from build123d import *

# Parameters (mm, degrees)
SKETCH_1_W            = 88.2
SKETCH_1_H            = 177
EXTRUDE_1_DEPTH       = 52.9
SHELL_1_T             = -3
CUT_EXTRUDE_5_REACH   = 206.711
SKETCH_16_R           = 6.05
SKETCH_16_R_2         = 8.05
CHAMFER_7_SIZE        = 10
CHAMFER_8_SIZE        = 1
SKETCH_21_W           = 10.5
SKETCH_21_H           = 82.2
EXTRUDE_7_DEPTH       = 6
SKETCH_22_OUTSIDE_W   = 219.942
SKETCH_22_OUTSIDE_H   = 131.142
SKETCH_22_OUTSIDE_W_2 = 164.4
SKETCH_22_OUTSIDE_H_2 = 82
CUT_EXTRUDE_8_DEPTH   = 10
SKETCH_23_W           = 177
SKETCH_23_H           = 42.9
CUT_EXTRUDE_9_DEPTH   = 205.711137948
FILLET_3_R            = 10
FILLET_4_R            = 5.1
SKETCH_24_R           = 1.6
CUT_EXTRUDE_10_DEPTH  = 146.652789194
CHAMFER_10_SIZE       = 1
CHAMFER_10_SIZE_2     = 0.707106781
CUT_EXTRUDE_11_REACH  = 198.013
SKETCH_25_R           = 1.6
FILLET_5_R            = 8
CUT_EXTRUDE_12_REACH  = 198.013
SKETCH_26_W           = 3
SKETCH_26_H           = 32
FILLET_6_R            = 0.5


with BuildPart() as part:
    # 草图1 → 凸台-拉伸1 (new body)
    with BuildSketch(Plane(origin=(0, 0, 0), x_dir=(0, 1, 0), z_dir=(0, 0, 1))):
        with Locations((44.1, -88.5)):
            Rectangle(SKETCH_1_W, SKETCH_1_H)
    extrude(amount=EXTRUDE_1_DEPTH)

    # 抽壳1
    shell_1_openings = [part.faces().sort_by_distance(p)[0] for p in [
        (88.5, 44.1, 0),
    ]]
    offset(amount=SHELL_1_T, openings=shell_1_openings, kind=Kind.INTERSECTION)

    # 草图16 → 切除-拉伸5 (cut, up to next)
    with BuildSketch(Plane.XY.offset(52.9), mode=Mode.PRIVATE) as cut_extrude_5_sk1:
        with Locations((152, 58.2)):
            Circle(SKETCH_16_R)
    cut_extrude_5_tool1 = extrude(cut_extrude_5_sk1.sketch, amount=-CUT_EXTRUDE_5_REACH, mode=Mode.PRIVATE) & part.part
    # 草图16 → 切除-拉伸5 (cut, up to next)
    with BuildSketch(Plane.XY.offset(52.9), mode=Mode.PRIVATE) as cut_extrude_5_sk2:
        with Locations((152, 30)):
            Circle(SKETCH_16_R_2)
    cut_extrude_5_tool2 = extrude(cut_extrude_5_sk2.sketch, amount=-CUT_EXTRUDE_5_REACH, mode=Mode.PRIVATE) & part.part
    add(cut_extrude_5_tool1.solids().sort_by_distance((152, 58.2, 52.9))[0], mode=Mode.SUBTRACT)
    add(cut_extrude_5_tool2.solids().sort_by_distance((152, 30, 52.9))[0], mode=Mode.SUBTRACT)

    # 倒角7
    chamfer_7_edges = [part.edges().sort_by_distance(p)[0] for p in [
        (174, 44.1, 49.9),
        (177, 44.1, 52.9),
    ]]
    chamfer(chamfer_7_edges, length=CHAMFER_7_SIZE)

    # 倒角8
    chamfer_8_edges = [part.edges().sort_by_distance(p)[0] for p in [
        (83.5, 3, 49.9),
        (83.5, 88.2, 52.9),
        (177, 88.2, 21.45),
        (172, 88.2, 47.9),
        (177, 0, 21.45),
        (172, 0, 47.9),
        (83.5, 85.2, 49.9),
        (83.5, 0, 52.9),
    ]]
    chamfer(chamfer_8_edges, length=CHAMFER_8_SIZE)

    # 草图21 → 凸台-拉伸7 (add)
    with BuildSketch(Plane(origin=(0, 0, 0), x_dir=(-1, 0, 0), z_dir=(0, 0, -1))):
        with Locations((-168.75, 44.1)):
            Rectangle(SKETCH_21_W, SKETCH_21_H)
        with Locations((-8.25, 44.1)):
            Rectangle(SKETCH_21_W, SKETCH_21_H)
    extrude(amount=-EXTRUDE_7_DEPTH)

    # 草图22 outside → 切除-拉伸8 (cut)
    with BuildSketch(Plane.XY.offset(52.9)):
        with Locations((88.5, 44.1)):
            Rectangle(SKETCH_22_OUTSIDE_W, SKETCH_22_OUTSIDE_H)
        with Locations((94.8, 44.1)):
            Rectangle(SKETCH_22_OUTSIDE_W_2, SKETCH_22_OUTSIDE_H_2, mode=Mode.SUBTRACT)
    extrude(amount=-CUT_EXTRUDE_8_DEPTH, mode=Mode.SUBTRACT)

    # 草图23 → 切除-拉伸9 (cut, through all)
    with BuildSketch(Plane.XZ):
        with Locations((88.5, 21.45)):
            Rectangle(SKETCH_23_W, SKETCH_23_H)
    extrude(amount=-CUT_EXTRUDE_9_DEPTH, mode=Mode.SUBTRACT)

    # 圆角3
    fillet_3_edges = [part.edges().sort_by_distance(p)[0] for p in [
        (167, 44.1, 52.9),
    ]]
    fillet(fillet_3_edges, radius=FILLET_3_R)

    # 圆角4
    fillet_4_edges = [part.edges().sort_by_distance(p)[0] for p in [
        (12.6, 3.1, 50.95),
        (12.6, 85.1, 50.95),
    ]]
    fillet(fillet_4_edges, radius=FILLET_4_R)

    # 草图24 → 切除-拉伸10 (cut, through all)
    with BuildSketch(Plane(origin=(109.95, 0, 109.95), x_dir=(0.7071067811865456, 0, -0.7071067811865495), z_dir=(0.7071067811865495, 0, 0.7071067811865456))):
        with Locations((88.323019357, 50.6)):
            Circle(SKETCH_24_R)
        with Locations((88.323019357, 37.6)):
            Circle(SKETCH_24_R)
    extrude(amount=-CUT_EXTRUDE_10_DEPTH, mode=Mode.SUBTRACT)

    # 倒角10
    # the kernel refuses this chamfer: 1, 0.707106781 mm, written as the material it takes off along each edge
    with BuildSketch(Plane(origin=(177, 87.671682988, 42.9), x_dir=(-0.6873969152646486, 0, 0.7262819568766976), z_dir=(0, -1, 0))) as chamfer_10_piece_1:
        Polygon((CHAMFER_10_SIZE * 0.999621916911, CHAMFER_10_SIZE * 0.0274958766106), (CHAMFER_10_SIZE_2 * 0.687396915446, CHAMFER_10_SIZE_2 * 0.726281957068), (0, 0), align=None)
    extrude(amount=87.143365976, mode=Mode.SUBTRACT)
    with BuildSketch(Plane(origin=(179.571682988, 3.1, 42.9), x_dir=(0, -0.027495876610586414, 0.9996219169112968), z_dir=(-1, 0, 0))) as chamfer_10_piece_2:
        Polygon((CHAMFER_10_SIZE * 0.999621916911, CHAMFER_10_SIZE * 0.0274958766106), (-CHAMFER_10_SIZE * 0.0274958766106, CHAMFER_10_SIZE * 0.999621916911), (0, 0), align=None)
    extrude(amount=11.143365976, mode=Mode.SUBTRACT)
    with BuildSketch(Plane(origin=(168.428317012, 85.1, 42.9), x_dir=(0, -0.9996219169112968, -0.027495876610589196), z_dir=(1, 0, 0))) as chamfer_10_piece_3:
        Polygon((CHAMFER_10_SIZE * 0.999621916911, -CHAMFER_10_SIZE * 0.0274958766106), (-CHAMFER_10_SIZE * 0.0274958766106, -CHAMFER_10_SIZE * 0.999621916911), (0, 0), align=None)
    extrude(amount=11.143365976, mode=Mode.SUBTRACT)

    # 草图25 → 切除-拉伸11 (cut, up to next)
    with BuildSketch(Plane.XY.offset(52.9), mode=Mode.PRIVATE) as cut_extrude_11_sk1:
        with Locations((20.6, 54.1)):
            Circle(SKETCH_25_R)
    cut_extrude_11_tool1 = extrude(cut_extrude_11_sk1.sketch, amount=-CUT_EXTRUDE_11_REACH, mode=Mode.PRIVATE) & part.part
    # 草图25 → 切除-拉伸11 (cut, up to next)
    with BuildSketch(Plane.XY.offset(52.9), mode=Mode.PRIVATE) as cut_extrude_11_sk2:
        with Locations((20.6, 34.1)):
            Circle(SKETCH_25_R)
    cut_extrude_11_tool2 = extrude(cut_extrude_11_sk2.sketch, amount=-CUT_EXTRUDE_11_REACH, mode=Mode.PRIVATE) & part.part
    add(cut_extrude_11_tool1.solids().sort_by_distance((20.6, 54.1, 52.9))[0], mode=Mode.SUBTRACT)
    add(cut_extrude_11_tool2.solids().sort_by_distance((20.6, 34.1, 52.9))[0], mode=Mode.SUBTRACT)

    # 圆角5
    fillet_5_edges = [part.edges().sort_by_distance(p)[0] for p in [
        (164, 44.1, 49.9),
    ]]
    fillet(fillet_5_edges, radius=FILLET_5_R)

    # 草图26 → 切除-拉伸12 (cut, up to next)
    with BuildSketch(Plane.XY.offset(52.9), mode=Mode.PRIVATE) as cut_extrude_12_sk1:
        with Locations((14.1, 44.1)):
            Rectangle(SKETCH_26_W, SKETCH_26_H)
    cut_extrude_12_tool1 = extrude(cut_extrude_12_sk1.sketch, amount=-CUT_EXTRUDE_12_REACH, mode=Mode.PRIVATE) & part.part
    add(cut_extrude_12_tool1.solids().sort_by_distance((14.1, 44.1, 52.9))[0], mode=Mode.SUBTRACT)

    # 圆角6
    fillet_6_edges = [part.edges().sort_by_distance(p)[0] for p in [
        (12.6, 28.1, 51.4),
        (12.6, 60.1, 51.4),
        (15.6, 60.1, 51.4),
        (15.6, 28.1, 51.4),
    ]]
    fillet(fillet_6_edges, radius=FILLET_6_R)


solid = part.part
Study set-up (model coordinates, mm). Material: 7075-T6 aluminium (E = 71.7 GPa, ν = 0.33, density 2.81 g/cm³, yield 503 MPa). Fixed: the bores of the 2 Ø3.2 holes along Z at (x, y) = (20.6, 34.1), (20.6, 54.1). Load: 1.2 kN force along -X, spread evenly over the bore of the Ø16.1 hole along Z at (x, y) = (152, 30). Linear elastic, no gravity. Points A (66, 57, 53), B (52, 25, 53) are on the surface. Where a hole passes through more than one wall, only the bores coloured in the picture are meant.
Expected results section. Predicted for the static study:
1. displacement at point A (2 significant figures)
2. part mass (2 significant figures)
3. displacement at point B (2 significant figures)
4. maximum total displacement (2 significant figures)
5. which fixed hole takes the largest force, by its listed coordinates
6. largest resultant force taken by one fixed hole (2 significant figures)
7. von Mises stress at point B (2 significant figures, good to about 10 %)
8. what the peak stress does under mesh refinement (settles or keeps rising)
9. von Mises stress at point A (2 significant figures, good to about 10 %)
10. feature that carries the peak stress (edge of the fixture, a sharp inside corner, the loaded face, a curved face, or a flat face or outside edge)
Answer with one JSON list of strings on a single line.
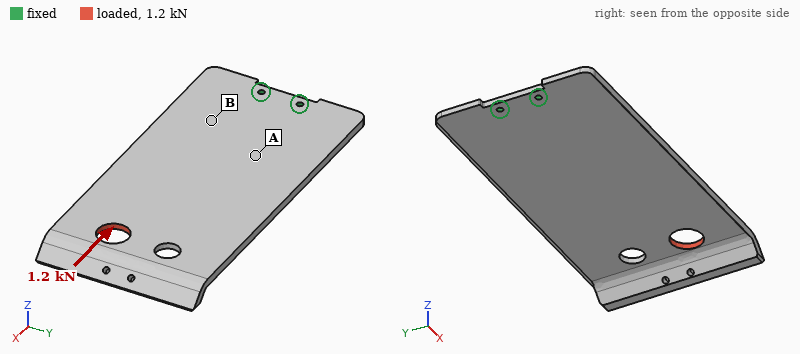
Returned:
["20 µm", "110 g", "19 µm", "88 µm", "(20.6, 34.1)", "1.4 kN", "10 MPa", "keeps rising", "4.1 MPa", "edge of the fixture"]
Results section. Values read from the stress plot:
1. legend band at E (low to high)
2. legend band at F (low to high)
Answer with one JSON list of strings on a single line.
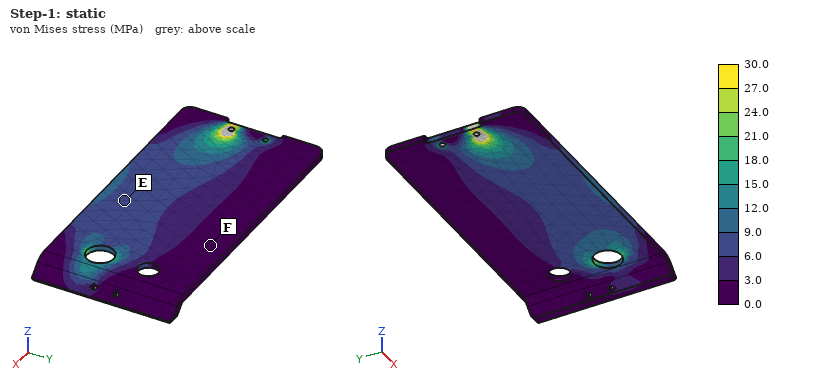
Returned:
["6.0 to 9.0 MPa", "0.0 to 3.0 MPa"]
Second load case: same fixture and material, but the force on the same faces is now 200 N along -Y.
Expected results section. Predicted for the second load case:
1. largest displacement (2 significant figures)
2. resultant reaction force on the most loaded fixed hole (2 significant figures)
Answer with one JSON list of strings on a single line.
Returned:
["0.13 mm", "1.2 kN"]
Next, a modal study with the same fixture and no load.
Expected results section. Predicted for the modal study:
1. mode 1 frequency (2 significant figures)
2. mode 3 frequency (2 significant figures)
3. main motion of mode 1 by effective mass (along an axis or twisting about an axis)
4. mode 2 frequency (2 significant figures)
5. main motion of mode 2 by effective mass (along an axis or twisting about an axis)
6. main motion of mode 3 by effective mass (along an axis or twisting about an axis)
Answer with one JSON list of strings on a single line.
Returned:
["92 Hz", "570 Hz", "along Z", "350 Hz", "twisting about X", "along Z"]
